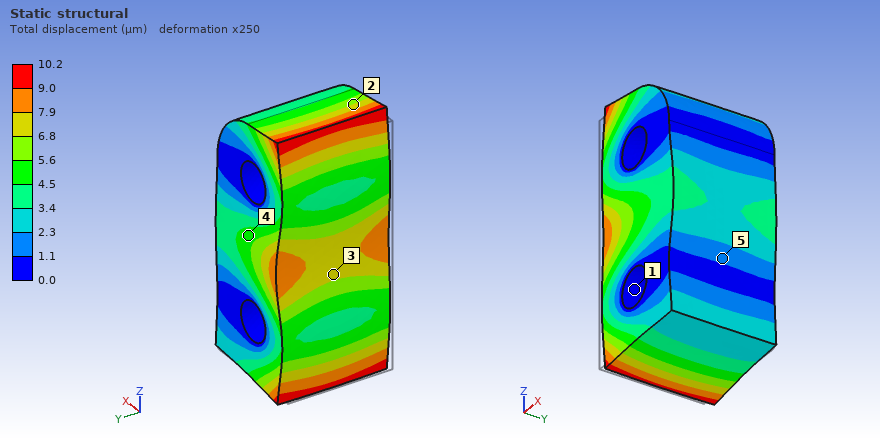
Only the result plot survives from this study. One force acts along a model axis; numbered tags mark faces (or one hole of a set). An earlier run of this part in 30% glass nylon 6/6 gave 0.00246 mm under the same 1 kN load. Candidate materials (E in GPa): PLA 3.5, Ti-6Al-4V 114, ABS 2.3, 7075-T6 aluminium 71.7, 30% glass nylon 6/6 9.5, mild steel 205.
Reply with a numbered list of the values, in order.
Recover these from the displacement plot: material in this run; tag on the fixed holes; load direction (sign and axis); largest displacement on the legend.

1. ABS
2. 1
3. +X
4. 10.2 µm
